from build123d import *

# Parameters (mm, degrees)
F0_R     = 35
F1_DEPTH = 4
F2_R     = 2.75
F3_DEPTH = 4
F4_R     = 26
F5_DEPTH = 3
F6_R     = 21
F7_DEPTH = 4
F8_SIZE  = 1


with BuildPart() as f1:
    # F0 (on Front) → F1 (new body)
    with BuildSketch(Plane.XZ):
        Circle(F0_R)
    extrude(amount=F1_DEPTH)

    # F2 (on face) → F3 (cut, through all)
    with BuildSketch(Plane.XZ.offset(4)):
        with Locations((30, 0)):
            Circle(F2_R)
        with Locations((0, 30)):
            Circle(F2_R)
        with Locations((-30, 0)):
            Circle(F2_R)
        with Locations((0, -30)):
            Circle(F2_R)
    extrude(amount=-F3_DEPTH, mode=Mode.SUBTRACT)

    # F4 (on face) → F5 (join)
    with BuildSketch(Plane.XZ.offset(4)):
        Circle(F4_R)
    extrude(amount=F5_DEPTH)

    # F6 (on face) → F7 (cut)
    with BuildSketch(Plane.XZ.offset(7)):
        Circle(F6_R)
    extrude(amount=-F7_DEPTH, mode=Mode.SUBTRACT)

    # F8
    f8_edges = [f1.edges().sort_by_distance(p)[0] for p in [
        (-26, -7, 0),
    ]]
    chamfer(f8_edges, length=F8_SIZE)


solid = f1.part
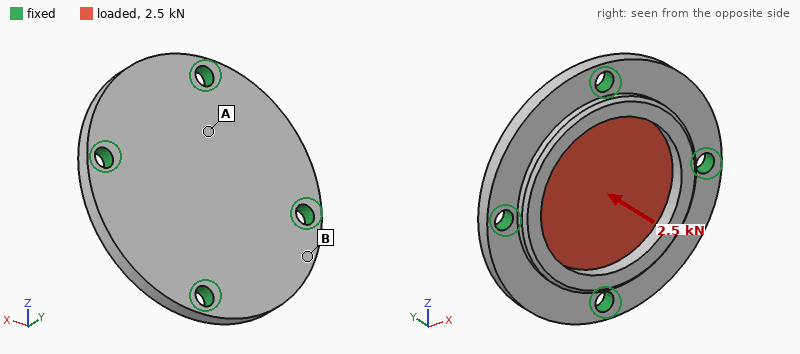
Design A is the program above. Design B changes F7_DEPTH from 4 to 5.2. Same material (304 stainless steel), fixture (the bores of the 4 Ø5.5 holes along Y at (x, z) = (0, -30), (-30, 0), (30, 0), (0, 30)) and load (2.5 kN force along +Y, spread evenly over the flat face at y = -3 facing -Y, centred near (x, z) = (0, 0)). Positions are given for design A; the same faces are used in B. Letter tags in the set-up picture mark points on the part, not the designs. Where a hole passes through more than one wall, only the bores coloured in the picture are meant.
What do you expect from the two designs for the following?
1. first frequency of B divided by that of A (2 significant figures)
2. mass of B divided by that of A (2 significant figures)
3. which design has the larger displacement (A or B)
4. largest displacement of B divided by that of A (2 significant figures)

0.86
0.89
B
2.6
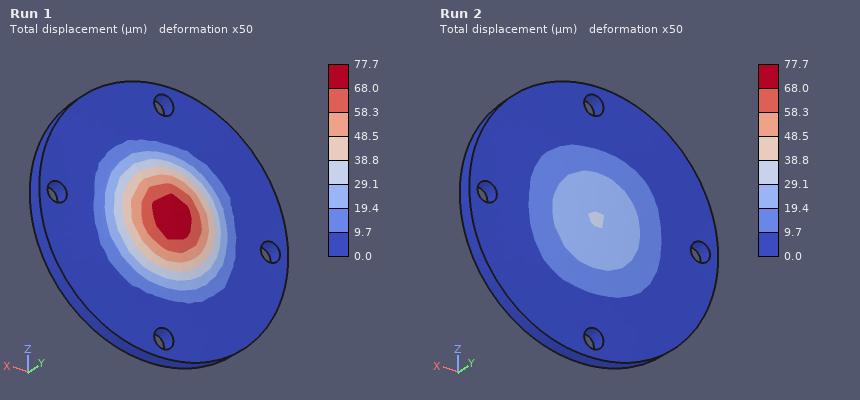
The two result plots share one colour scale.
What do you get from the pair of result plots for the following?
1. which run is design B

Run 1
